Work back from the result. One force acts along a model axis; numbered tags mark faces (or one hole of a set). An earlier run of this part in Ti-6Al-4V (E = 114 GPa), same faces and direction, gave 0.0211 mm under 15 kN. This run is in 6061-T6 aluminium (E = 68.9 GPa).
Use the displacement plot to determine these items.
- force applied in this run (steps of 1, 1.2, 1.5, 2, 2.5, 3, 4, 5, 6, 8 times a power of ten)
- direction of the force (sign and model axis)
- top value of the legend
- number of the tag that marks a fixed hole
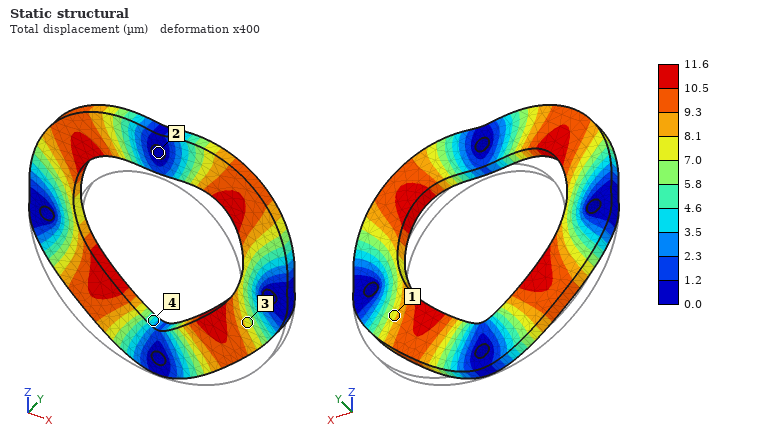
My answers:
5 kN
+Z
11.6 µm
2
